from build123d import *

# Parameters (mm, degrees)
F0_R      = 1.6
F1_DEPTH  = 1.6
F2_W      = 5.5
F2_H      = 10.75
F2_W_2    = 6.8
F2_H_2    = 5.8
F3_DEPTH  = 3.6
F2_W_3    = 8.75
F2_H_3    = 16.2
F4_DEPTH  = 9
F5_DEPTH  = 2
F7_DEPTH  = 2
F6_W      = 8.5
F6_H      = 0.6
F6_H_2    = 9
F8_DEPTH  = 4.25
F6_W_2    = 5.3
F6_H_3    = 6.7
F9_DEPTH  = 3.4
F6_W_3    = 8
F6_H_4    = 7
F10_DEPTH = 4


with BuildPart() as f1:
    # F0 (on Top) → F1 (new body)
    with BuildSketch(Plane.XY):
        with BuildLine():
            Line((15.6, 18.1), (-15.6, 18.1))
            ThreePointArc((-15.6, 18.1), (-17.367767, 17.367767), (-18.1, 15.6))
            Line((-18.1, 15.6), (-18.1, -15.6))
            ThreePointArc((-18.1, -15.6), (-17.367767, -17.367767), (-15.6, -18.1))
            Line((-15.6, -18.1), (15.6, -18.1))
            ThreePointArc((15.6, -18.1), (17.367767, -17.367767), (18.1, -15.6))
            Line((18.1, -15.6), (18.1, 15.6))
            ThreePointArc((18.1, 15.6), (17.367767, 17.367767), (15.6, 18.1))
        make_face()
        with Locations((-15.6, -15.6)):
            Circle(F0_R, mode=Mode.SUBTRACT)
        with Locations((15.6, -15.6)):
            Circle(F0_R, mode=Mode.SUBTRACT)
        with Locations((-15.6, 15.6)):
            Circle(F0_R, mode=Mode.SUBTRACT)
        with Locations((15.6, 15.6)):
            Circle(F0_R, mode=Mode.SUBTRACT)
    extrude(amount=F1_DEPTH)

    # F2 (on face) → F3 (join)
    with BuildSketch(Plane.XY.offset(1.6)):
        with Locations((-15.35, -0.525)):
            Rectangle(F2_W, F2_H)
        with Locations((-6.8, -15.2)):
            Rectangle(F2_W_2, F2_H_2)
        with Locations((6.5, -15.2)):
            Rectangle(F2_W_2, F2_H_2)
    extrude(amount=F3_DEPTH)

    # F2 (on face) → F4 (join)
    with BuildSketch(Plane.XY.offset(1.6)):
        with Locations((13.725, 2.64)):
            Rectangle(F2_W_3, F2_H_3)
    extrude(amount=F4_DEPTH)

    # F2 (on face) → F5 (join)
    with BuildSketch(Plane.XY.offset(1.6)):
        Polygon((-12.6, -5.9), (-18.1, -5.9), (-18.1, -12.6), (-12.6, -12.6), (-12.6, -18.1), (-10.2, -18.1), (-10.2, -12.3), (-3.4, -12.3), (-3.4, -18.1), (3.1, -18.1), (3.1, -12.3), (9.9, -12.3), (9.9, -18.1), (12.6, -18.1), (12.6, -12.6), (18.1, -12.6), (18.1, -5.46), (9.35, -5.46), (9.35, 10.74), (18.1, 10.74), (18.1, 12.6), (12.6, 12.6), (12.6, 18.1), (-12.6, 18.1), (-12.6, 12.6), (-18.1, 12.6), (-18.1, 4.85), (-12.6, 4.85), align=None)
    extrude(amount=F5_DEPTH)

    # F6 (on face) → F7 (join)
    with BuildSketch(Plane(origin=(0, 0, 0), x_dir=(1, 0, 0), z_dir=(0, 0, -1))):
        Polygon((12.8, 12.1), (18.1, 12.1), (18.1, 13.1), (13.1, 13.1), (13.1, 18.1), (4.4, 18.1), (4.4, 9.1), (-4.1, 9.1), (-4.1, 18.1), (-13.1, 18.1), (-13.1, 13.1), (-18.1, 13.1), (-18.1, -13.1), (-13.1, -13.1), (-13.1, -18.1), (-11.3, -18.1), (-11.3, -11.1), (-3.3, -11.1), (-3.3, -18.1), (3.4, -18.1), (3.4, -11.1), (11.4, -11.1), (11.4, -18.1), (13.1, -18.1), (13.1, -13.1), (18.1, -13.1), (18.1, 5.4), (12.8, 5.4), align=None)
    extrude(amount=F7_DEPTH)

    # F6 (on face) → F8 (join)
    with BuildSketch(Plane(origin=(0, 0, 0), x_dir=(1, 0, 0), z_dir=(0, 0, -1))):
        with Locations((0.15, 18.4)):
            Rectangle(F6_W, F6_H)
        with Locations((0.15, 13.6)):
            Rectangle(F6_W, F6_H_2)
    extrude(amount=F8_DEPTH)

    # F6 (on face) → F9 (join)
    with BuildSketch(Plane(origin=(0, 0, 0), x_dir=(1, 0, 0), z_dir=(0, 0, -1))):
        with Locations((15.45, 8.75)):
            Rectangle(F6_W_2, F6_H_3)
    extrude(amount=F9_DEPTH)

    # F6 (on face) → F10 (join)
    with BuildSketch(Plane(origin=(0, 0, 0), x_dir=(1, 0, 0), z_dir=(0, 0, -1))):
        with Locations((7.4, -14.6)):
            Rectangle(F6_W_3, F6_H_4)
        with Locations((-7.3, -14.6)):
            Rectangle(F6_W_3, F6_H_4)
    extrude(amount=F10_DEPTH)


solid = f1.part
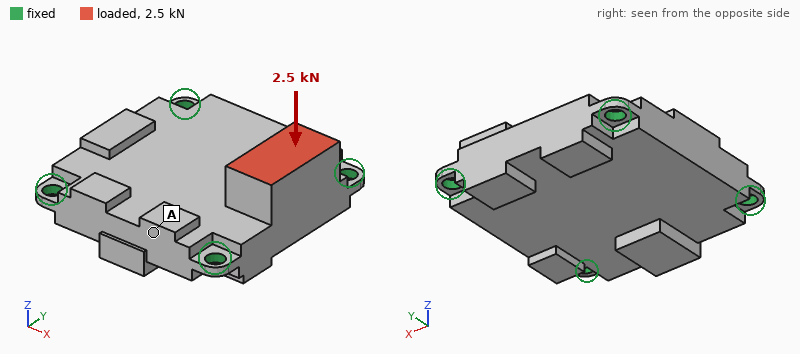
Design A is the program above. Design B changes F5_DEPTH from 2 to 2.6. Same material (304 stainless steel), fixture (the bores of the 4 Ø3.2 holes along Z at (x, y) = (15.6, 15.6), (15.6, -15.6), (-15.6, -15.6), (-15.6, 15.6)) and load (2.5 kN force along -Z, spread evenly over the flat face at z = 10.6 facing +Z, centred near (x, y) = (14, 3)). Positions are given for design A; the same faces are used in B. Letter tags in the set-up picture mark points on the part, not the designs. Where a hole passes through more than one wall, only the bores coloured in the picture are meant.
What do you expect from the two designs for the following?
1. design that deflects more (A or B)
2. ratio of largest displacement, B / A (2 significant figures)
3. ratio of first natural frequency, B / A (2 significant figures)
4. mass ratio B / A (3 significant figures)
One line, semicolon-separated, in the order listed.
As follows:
A; 0.88; 1.1; 1.06
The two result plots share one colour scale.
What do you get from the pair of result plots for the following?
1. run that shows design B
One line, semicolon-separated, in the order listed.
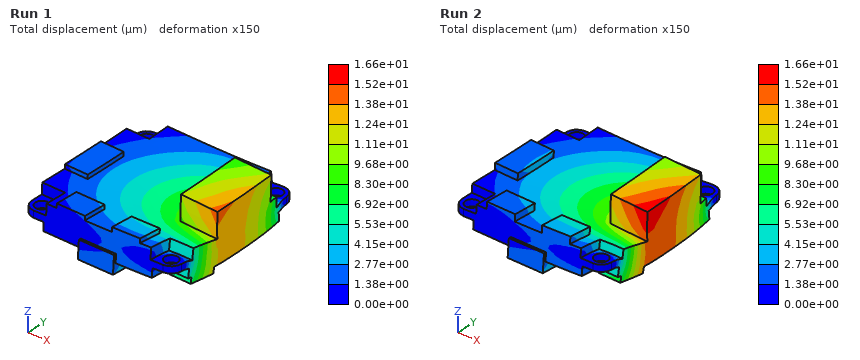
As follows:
Run 1
